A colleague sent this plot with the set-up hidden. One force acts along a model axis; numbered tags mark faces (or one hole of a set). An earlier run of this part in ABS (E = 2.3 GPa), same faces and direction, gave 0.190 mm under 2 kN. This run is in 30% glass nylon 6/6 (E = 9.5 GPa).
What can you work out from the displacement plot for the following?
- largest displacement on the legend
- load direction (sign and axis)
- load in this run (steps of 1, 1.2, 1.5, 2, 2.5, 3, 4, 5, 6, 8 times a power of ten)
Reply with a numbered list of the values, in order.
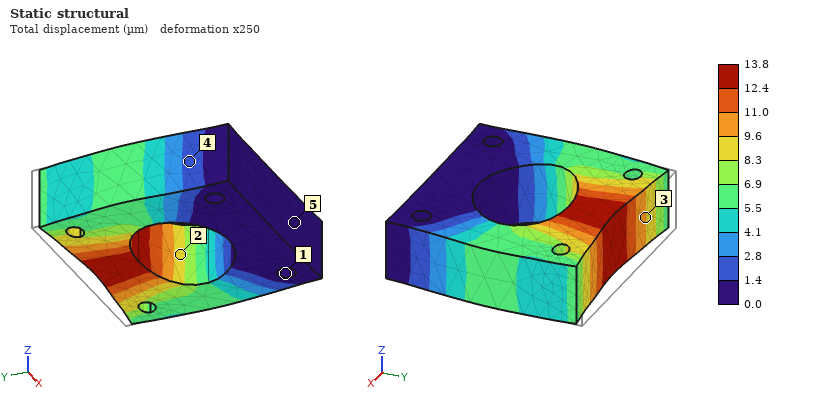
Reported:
1. 13.8 µm
2. -Y
3. 600 N
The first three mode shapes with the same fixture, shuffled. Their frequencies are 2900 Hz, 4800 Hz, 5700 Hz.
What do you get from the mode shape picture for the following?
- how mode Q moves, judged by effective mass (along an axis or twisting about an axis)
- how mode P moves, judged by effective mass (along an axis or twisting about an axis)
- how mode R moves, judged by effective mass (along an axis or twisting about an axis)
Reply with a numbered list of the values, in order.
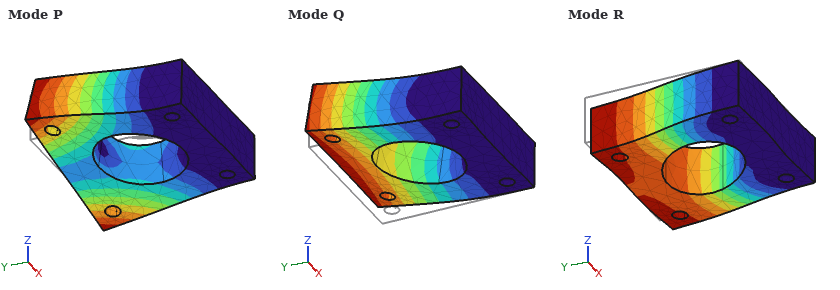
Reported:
1. along Z
2. twisting about Y
3. along X
